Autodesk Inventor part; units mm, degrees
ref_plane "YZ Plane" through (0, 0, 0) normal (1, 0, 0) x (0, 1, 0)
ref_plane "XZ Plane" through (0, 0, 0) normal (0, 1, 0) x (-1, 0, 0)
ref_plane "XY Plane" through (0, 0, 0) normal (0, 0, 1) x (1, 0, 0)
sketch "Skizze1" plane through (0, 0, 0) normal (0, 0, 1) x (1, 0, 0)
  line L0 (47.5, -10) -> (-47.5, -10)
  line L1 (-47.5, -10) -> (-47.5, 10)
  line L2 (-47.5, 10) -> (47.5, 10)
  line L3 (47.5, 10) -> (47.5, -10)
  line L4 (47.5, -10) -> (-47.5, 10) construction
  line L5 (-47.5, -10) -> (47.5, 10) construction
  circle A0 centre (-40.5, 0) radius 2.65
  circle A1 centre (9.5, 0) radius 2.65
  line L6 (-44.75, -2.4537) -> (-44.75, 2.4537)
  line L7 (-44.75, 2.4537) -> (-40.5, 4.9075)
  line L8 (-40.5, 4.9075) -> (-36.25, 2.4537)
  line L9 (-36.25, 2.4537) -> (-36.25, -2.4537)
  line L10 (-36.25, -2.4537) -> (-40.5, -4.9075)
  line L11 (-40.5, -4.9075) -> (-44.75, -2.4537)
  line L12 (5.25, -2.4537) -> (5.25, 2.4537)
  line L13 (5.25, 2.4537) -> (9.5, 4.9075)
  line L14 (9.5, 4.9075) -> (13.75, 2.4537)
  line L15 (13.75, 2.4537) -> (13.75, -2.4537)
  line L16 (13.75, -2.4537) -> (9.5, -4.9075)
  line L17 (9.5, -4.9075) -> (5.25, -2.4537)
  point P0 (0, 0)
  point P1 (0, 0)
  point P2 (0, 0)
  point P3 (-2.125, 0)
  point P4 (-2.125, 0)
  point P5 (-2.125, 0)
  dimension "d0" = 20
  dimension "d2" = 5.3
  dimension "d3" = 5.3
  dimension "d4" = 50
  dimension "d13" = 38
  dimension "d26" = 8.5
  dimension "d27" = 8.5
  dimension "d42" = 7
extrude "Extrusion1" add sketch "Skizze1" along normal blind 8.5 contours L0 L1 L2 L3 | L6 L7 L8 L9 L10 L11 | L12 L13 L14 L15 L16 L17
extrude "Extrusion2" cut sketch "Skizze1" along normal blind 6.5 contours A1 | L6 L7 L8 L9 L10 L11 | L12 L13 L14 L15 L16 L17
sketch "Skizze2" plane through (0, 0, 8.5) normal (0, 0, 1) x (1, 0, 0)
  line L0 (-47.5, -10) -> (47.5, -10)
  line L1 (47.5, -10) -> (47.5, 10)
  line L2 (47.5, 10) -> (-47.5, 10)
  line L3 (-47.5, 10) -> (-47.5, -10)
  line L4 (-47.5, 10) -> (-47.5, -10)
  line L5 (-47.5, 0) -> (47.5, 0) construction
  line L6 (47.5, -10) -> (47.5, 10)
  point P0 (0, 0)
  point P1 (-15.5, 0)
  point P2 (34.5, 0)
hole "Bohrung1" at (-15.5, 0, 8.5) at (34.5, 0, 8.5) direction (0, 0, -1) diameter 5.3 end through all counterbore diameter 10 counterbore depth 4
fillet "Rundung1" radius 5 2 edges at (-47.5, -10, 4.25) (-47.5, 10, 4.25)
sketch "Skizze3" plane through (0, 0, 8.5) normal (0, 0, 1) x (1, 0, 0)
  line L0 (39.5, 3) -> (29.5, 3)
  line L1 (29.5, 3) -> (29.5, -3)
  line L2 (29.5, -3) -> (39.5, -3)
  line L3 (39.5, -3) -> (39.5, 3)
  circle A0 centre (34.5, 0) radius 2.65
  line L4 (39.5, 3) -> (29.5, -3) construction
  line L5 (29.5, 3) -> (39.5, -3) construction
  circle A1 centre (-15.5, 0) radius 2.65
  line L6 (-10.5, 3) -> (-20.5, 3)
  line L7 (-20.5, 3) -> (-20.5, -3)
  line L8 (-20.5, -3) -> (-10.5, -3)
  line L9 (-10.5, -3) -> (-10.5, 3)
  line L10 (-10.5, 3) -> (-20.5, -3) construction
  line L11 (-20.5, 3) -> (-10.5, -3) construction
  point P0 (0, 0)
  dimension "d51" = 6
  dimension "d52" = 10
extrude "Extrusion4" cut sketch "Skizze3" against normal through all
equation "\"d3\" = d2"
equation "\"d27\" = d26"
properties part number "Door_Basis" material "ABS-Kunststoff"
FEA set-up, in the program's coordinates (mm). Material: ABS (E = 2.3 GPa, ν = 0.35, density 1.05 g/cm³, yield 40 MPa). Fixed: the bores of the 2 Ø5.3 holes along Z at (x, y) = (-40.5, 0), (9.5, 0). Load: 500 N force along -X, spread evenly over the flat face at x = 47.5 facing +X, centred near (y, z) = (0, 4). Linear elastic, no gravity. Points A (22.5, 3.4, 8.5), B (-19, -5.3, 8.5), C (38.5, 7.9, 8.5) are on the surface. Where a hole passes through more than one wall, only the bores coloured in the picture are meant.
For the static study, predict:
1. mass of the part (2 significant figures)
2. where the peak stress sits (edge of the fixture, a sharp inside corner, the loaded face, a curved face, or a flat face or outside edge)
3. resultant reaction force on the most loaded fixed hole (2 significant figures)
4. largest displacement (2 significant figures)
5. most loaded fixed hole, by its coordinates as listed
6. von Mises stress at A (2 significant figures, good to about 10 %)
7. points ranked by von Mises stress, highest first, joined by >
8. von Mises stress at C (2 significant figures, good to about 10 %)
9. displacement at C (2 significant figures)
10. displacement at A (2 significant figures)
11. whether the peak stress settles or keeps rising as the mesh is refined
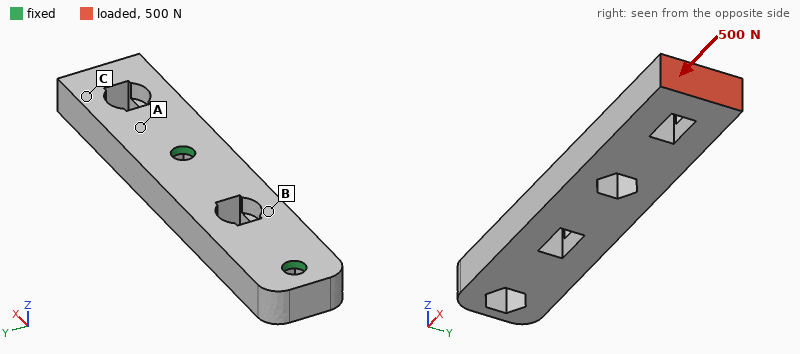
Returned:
15 g
edge of the fixture
350 N
0.29 mm
(9.5, 0)
2.8 MPa
C > A > B
5.1 MPa
0.21 mm
0.090 mm
keeps rising
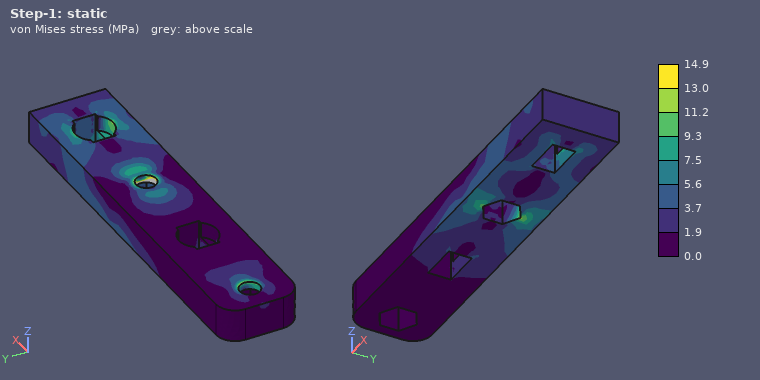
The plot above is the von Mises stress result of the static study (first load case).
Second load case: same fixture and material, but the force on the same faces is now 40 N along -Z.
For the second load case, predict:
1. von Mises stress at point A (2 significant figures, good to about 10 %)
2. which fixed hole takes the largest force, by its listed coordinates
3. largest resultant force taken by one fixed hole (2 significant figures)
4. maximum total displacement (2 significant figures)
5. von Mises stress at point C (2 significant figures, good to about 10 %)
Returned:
4.0 MPa
(9.5, 0)
110 N
0.61 mm
2.6 MPa
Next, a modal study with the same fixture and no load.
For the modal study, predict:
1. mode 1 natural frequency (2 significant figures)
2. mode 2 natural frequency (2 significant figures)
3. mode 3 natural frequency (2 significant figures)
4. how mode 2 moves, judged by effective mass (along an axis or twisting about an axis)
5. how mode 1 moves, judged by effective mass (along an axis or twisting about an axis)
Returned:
1000 Hz
1600 Hz
2100 Hz
along Y
along Z
